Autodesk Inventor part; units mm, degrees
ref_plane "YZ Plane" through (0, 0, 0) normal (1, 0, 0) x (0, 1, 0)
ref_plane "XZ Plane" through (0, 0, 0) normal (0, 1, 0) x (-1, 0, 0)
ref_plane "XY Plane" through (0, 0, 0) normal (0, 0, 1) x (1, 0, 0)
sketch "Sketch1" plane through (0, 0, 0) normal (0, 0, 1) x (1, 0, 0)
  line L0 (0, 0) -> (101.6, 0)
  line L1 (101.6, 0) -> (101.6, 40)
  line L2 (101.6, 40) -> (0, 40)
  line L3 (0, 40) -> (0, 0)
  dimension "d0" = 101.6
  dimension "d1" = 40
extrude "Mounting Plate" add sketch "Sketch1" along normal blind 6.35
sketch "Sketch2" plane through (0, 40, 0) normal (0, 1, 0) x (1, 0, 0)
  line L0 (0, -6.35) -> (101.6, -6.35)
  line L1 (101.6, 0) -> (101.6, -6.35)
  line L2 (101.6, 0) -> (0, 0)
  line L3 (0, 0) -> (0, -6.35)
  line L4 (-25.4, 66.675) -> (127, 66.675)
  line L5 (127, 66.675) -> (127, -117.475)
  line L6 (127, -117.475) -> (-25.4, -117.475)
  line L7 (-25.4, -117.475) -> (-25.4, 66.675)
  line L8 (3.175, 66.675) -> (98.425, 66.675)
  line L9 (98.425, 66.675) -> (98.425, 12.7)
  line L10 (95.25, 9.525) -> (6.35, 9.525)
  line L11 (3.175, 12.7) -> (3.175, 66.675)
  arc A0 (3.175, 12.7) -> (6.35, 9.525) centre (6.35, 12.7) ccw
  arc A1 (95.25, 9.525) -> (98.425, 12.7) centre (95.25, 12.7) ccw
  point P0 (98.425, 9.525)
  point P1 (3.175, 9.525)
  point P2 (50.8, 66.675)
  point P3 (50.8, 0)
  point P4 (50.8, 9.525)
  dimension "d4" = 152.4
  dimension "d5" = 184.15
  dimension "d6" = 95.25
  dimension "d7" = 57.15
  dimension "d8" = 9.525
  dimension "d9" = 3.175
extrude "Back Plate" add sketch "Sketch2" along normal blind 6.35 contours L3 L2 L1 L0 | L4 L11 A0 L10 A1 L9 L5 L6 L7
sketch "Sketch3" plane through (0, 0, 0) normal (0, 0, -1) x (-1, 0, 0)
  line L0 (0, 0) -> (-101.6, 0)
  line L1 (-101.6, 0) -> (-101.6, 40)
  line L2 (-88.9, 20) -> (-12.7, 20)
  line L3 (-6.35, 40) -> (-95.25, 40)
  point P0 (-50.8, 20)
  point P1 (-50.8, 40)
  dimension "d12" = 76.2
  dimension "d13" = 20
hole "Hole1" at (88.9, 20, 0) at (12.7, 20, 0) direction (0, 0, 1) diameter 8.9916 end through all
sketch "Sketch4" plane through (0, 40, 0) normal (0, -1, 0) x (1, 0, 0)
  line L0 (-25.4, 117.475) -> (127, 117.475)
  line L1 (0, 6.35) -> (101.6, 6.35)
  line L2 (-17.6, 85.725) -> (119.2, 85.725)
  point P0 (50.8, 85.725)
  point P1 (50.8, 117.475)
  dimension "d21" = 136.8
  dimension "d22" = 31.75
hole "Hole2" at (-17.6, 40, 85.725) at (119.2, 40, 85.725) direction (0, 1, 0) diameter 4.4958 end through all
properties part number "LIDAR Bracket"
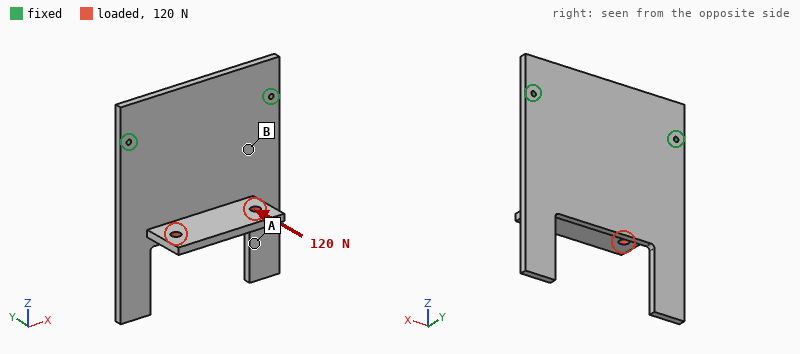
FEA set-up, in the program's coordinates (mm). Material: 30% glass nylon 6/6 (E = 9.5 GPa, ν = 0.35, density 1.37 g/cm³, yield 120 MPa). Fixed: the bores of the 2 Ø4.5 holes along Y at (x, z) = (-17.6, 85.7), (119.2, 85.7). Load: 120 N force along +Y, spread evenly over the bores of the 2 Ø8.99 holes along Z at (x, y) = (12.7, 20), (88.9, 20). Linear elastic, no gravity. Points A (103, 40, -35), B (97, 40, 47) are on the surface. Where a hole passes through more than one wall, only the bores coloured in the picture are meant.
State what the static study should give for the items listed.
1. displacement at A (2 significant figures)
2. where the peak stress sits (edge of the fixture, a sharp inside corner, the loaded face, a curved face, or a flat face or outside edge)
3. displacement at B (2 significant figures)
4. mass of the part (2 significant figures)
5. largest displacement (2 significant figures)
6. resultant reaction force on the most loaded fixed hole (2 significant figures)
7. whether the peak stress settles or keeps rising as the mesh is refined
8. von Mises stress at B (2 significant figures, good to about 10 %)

2.1 mm
edge of the fixture
0.49 mm
230 g
2.8 mm
60 N
keeps rising
5.5 MPa
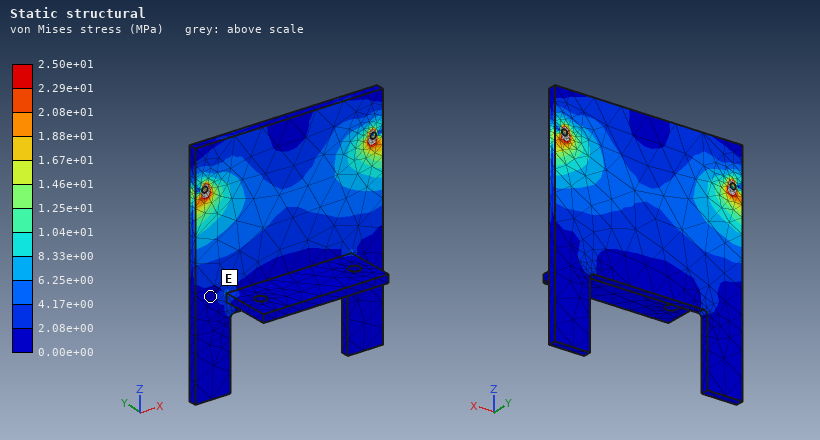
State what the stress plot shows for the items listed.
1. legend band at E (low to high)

0.00e+00 to 2.08e+00 MPa
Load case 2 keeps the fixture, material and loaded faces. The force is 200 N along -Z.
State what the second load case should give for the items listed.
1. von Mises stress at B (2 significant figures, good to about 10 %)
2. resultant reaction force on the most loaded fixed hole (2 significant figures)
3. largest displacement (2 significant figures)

4.6 MPa
100 N
1.8 mm
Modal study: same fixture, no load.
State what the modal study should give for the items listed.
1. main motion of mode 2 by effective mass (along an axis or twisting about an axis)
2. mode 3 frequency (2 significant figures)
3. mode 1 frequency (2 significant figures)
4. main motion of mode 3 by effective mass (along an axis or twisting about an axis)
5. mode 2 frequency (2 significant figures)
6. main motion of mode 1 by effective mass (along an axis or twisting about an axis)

twisting about Z
550 Hz
110 Hz
along Y
250 Hz
along Y
